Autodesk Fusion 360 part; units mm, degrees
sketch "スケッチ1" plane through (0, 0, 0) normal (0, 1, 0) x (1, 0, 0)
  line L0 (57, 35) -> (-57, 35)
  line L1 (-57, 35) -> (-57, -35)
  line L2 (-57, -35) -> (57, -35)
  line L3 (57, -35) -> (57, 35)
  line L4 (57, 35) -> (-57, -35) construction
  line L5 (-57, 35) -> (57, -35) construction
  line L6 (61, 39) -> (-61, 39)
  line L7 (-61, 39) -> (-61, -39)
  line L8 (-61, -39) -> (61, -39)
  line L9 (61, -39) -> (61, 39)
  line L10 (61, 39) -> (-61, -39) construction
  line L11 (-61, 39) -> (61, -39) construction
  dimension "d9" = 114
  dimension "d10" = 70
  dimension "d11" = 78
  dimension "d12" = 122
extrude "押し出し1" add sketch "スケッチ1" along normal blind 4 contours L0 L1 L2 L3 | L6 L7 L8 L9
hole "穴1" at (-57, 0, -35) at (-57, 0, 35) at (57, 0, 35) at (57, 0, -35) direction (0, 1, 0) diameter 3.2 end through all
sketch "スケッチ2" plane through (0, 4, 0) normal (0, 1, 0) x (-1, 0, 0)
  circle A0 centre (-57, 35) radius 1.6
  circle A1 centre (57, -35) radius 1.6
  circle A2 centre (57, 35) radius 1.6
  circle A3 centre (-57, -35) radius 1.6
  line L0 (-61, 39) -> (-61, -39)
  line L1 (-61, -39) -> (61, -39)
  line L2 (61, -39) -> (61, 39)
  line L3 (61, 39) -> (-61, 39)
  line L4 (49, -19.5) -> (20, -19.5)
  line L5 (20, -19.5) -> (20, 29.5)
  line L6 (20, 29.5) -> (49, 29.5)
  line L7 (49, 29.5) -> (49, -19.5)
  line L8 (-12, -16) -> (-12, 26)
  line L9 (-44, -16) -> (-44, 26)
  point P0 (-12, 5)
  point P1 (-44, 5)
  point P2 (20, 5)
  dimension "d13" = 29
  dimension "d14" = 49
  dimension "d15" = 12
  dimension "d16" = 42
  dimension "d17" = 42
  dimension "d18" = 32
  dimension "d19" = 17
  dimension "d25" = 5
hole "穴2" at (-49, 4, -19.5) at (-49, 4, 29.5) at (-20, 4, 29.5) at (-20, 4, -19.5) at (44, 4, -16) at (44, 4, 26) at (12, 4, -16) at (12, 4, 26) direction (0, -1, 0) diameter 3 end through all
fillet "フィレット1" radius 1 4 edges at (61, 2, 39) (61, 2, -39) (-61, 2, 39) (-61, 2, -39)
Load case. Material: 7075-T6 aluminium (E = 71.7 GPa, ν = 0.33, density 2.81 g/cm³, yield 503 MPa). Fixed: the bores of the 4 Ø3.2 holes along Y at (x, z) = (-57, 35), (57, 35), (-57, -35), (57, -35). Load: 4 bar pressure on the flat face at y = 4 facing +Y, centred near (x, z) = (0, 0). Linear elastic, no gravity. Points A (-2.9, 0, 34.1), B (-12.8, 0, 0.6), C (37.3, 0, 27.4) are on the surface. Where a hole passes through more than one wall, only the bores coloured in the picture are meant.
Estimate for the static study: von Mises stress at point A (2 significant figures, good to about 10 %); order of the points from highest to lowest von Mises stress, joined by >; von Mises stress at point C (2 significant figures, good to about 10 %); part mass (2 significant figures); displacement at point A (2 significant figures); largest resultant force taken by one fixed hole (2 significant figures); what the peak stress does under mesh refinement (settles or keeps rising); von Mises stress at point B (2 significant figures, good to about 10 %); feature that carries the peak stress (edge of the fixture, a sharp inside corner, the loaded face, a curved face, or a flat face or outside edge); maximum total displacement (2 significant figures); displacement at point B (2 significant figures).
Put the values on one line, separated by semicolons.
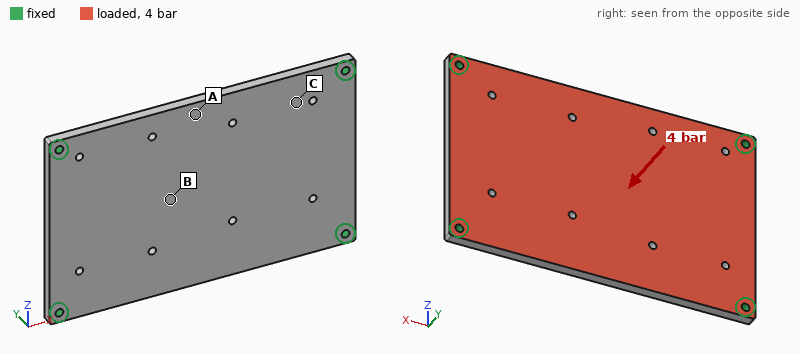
120 MPa; A > B > C; 34 MPa; 110 g; 0.78 mm; 940 N; keeps rising; 85 MPa; edge of the fixture; 0.81 mm; 0.76 mm
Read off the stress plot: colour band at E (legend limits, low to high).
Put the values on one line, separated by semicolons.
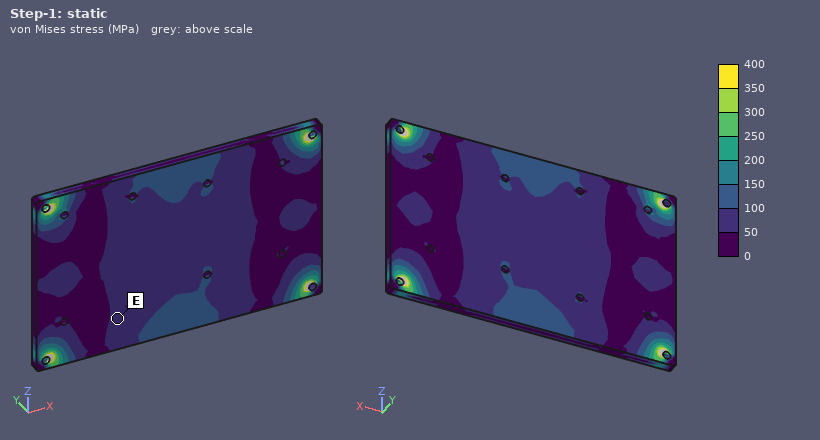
50 to 100 MPa
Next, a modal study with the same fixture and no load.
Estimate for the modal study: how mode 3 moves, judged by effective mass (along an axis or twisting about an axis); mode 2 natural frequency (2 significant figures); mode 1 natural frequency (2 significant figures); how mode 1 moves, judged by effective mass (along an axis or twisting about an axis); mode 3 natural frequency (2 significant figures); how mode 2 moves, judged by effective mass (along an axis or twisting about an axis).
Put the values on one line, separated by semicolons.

twisting about Z; 2100 Hz; 1200 Hz; along Y; 3100 Hz; twisting about X
